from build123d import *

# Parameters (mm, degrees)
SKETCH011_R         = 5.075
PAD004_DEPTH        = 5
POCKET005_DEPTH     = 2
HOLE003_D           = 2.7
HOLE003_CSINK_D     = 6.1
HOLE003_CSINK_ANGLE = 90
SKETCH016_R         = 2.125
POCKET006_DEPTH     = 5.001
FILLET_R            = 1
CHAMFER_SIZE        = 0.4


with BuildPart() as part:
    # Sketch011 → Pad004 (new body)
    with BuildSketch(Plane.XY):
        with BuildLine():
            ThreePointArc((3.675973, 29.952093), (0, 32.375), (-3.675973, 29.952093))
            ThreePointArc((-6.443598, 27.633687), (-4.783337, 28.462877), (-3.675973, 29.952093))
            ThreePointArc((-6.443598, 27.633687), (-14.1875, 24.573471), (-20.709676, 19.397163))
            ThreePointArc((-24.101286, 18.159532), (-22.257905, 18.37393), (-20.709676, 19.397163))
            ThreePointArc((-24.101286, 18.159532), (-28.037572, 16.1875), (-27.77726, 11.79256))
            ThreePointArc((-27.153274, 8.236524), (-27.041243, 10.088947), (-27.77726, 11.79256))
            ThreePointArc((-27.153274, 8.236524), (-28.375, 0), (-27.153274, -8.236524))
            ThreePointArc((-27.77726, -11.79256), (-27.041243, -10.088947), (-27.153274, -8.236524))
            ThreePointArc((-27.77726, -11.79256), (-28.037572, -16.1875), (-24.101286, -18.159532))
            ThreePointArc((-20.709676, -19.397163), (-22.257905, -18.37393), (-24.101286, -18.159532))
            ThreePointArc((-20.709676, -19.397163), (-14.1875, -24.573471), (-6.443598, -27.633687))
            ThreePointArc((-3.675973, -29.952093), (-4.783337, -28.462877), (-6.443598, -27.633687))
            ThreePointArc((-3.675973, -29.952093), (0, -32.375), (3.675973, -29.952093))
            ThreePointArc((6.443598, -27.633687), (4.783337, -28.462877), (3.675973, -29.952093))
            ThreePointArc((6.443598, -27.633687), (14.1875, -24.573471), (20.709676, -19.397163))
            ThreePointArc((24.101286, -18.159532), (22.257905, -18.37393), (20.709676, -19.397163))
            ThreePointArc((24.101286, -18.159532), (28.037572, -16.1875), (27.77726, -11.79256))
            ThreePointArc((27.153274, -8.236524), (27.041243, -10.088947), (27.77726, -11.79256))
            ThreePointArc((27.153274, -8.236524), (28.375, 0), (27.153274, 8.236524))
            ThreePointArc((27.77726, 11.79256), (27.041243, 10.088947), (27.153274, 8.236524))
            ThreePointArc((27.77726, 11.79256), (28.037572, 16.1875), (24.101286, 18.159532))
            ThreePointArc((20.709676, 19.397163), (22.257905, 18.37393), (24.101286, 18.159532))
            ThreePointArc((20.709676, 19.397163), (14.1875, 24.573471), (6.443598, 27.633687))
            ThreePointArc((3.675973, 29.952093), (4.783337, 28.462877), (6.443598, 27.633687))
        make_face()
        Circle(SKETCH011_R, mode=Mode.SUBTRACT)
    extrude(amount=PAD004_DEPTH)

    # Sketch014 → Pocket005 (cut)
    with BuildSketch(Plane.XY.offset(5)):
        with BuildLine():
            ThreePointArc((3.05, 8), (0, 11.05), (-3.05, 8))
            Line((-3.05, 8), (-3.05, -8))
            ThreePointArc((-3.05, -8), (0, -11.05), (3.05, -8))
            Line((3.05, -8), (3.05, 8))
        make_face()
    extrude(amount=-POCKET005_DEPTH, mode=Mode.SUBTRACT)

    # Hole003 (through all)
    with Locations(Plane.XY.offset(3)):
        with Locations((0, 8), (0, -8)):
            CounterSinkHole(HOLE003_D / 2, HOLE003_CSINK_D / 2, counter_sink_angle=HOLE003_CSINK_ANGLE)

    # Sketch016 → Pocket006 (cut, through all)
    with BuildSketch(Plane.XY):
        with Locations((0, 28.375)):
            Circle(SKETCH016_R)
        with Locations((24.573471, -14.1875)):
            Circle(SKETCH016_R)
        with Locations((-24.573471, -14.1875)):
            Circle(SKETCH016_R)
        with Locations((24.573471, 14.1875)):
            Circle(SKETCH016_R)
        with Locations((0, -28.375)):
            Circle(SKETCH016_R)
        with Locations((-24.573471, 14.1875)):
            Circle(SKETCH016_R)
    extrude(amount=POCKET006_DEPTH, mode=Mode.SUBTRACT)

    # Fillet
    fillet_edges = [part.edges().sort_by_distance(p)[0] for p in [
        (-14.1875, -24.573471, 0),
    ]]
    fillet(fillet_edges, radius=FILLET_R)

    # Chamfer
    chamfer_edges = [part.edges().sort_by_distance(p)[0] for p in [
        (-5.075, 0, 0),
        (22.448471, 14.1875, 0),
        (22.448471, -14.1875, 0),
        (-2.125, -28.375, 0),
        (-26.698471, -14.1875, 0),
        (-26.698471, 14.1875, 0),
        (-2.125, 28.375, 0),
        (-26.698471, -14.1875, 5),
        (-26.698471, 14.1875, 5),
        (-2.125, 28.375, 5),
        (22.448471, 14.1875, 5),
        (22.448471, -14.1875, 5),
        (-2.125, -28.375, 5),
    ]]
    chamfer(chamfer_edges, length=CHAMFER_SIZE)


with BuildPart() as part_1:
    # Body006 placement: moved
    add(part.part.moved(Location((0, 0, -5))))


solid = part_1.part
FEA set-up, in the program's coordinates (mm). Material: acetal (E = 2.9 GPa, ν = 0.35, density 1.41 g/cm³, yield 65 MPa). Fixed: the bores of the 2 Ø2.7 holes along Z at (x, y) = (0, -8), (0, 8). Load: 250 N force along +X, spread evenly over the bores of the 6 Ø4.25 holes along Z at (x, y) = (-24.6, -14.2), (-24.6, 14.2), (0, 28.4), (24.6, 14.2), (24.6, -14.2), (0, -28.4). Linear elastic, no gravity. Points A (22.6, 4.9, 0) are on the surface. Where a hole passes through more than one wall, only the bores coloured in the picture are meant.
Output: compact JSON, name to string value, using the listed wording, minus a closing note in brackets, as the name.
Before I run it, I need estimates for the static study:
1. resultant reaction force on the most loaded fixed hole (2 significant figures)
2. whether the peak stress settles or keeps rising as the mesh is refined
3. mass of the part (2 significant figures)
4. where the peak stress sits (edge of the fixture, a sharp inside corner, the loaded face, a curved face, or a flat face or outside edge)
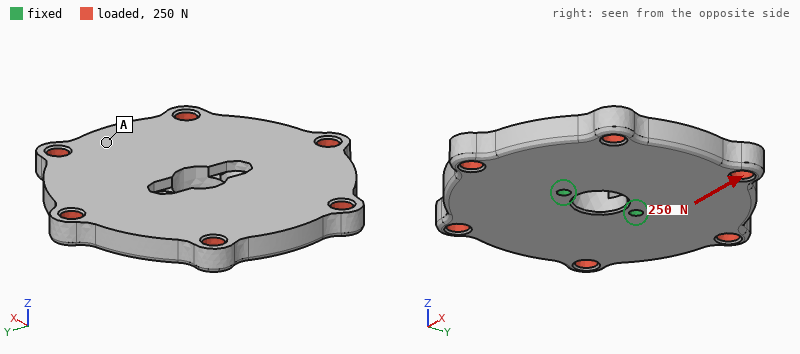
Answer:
{"resultant reaction force on the most loaded fixed hole": "130 N", "whether the peak stress settles or keeps rising as the mesh is refined": "keeps rising", "mass of the part": "17 g", "where the peak stress sits": "edge of the fixture"}
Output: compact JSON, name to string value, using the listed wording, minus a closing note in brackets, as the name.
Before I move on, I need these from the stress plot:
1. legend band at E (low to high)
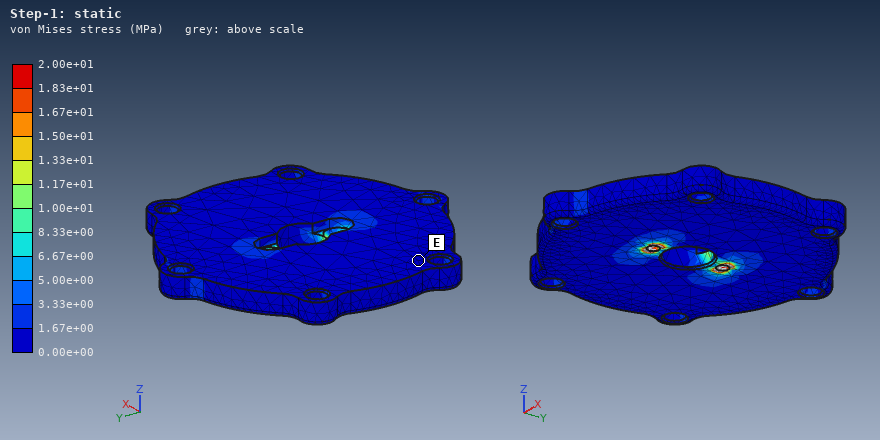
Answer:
{"legend band at E": "0.00e+00 to 1.67e+00 MPa"}
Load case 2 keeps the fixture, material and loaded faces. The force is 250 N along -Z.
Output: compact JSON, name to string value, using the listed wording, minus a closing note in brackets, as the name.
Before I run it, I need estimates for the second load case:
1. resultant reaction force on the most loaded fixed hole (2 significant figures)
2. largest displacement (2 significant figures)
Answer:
{"resultant reaction force on the most loaded fixed hole": "190 N", "largest displacement": "0.48 mm"}
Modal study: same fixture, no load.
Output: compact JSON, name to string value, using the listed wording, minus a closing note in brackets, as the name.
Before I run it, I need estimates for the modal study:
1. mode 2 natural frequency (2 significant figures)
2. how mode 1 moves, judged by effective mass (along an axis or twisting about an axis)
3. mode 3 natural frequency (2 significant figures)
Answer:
{"mode 2 natural frequency": "1400 Hz", "how mode 1 moves, judged by effective mass": "twisting about Y", "mode 3 natural frequency": "1400 Hz"}
